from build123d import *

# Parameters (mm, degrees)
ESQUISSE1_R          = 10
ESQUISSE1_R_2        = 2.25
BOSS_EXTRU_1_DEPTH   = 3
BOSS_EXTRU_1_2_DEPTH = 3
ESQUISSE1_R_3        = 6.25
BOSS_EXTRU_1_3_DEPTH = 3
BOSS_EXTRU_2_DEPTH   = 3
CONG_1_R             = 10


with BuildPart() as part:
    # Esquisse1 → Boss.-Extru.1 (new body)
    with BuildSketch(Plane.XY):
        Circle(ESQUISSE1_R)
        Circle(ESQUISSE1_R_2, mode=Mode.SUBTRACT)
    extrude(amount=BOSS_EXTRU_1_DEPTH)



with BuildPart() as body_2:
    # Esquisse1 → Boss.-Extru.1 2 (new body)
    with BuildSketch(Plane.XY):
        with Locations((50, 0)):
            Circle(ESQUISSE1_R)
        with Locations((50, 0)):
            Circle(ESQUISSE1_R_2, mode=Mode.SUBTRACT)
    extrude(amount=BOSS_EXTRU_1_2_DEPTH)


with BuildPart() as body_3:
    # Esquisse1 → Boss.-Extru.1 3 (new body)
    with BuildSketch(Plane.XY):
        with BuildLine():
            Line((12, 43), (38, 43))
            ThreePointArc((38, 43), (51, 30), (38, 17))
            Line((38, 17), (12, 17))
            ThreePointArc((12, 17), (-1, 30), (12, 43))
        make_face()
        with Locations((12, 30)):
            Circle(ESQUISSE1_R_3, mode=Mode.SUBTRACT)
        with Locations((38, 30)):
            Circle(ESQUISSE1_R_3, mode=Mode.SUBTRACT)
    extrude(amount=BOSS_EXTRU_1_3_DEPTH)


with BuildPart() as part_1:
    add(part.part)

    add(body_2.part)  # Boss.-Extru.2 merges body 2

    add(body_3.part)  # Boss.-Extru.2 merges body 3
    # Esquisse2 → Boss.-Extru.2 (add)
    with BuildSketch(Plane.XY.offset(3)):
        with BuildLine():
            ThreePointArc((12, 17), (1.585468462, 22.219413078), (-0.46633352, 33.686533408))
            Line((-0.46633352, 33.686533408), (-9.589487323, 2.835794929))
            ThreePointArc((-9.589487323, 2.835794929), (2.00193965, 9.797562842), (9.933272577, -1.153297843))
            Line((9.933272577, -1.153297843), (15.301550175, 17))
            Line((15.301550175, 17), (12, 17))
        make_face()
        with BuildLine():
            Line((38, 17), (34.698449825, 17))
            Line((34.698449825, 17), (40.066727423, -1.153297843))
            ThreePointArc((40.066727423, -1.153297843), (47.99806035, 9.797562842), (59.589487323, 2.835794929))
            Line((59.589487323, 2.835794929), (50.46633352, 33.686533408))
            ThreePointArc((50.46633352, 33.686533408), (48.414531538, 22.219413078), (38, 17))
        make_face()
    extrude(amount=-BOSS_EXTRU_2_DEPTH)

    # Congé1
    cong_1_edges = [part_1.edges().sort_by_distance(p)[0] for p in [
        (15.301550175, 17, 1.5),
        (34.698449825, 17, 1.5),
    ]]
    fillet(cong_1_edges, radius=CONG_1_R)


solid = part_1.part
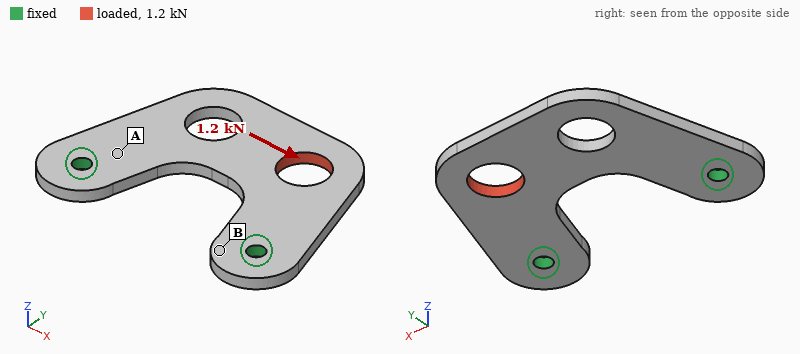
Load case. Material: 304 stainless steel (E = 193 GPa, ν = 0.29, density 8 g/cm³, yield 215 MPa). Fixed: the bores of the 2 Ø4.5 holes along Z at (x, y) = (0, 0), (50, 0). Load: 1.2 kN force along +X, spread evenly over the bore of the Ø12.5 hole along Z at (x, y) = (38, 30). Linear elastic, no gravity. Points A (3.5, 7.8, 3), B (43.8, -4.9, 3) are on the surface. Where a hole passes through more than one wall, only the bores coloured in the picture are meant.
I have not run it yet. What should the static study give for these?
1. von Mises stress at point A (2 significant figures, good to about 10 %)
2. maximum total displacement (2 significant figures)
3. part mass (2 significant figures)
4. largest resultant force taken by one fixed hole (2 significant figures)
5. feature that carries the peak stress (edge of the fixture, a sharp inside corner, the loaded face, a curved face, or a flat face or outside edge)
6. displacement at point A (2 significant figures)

24 MPa
11 µm
51 g
840 N
edge of the fixture
2.4 µm
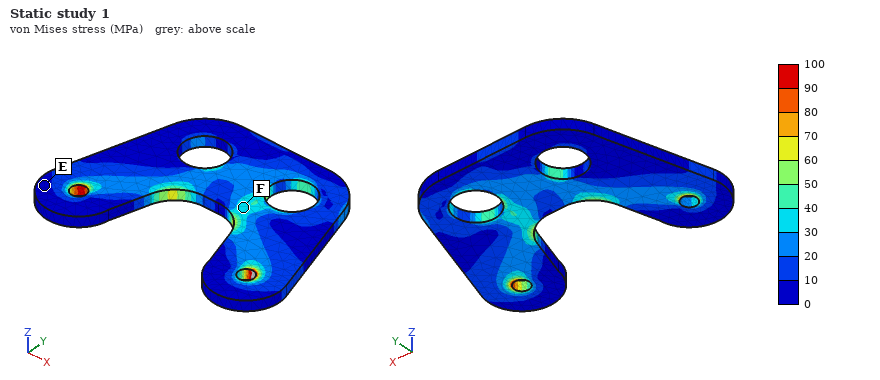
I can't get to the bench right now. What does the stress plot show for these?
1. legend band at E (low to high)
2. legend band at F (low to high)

0 to 10 MPa
30 to 40 MPa
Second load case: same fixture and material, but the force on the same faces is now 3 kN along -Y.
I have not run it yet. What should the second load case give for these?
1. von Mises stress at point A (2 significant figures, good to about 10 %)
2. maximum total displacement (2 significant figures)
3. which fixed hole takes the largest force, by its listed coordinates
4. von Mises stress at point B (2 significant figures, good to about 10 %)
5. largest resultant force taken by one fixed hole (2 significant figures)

25 MPa
11 µm
(50, 0)
18 MPa
2.4 kN
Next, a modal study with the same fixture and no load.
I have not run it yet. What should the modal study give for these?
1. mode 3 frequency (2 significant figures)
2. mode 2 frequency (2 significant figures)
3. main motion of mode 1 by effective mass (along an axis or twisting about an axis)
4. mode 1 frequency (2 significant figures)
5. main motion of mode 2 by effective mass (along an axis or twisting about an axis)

6200 Hz
3200 Hz
along Z
1300 Hz
twisting about Y
